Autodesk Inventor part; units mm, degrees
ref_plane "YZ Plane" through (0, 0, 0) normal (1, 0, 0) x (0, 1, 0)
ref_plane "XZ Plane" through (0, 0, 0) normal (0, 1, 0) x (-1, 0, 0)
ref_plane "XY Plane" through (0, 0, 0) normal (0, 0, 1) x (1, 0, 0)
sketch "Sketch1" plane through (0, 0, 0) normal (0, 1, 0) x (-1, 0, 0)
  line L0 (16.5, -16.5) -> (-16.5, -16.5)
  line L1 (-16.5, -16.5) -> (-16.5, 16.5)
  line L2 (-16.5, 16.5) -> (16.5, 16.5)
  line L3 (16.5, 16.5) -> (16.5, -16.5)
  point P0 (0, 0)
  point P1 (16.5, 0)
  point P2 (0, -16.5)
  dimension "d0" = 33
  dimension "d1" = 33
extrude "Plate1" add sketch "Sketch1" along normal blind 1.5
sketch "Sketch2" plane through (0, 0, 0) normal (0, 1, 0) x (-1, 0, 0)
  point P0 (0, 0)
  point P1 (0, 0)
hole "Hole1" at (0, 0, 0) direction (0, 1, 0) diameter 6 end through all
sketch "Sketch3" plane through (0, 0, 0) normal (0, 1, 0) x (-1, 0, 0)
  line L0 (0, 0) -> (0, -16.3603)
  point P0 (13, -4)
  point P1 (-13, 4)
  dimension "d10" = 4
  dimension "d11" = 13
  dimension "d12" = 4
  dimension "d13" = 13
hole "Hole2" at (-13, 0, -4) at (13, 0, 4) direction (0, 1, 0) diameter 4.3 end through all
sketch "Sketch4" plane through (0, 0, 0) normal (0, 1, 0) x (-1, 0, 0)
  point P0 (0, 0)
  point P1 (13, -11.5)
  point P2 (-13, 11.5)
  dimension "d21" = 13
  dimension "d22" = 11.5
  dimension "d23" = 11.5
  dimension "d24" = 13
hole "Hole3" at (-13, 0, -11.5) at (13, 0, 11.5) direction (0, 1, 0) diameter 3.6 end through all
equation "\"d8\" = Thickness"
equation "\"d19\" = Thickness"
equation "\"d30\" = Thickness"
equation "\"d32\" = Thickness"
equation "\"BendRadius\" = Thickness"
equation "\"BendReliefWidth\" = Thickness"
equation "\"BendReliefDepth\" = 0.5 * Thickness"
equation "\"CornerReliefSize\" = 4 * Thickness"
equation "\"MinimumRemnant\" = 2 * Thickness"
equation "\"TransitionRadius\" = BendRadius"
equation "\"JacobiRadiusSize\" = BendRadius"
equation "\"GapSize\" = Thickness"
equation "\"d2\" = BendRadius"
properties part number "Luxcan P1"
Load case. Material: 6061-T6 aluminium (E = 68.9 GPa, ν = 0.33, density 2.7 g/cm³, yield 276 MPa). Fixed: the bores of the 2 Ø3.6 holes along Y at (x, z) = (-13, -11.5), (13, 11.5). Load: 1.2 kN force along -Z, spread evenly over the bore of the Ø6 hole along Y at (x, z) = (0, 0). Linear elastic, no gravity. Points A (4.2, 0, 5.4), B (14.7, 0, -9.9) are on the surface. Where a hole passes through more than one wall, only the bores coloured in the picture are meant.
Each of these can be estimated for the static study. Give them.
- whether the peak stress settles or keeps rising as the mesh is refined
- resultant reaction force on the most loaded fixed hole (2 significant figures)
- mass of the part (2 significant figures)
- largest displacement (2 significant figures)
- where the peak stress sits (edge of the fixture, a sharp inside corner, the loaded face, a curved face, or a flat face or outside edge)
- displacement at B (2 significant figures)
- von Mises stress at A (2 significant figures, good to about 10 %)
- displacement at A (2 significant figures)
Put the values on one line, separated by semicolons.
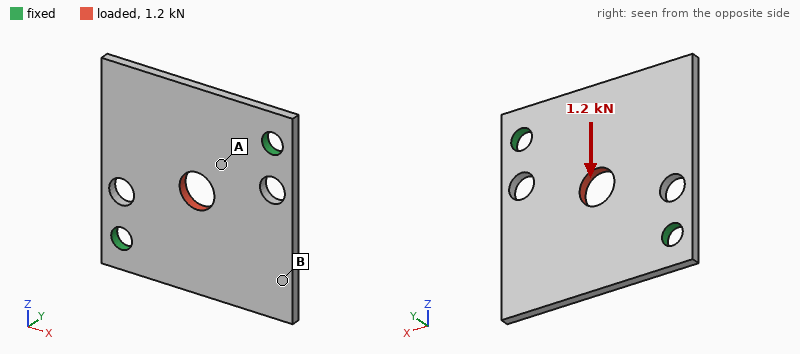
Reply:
keeps rising; 600 N; 4.1 g; 15 µm; edge of the fixture; 10.0 µm; 31 MPa; 11 µm
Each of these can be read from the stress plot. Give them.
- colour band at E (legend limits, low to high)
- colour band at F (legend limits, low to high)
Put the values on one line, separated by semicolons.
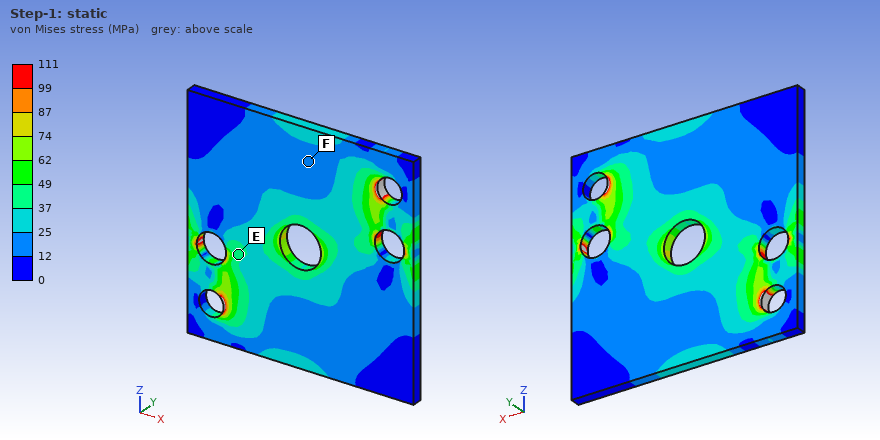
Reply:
37 to 49 MPa; 12 to 25 MPa
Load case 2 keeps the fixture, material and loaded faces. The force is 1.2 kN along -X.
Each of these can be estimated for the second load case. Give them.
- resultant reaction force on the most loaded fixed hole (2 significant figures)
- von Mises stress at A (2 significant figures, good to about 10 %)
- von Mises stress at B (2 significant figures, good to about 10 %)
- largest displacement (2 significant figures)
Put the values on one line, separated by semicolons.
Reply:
600 N; 37 MPa; 8.0 MPa; 13 µm
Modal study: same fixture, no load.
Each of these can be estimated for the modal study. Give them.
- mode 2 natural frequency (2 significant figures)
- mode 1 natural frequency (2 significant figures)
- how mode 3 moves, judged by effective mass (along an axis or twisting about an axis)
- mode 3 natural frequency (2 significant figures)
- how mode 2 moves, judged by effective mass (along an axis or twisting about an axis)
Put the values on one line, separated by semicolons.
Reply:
3300 Hz; 2600 Hz; along Y; 8800 Hz; along Y
